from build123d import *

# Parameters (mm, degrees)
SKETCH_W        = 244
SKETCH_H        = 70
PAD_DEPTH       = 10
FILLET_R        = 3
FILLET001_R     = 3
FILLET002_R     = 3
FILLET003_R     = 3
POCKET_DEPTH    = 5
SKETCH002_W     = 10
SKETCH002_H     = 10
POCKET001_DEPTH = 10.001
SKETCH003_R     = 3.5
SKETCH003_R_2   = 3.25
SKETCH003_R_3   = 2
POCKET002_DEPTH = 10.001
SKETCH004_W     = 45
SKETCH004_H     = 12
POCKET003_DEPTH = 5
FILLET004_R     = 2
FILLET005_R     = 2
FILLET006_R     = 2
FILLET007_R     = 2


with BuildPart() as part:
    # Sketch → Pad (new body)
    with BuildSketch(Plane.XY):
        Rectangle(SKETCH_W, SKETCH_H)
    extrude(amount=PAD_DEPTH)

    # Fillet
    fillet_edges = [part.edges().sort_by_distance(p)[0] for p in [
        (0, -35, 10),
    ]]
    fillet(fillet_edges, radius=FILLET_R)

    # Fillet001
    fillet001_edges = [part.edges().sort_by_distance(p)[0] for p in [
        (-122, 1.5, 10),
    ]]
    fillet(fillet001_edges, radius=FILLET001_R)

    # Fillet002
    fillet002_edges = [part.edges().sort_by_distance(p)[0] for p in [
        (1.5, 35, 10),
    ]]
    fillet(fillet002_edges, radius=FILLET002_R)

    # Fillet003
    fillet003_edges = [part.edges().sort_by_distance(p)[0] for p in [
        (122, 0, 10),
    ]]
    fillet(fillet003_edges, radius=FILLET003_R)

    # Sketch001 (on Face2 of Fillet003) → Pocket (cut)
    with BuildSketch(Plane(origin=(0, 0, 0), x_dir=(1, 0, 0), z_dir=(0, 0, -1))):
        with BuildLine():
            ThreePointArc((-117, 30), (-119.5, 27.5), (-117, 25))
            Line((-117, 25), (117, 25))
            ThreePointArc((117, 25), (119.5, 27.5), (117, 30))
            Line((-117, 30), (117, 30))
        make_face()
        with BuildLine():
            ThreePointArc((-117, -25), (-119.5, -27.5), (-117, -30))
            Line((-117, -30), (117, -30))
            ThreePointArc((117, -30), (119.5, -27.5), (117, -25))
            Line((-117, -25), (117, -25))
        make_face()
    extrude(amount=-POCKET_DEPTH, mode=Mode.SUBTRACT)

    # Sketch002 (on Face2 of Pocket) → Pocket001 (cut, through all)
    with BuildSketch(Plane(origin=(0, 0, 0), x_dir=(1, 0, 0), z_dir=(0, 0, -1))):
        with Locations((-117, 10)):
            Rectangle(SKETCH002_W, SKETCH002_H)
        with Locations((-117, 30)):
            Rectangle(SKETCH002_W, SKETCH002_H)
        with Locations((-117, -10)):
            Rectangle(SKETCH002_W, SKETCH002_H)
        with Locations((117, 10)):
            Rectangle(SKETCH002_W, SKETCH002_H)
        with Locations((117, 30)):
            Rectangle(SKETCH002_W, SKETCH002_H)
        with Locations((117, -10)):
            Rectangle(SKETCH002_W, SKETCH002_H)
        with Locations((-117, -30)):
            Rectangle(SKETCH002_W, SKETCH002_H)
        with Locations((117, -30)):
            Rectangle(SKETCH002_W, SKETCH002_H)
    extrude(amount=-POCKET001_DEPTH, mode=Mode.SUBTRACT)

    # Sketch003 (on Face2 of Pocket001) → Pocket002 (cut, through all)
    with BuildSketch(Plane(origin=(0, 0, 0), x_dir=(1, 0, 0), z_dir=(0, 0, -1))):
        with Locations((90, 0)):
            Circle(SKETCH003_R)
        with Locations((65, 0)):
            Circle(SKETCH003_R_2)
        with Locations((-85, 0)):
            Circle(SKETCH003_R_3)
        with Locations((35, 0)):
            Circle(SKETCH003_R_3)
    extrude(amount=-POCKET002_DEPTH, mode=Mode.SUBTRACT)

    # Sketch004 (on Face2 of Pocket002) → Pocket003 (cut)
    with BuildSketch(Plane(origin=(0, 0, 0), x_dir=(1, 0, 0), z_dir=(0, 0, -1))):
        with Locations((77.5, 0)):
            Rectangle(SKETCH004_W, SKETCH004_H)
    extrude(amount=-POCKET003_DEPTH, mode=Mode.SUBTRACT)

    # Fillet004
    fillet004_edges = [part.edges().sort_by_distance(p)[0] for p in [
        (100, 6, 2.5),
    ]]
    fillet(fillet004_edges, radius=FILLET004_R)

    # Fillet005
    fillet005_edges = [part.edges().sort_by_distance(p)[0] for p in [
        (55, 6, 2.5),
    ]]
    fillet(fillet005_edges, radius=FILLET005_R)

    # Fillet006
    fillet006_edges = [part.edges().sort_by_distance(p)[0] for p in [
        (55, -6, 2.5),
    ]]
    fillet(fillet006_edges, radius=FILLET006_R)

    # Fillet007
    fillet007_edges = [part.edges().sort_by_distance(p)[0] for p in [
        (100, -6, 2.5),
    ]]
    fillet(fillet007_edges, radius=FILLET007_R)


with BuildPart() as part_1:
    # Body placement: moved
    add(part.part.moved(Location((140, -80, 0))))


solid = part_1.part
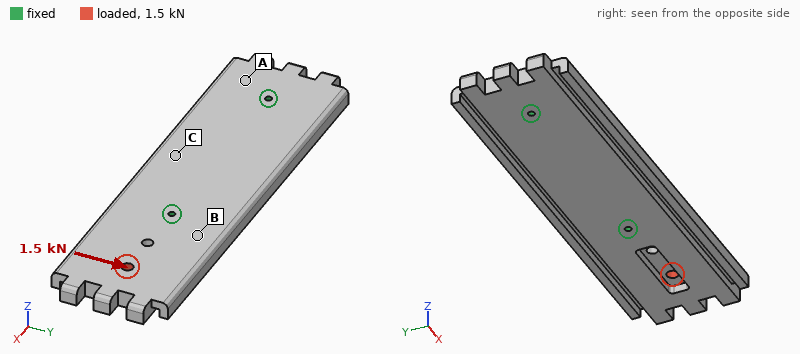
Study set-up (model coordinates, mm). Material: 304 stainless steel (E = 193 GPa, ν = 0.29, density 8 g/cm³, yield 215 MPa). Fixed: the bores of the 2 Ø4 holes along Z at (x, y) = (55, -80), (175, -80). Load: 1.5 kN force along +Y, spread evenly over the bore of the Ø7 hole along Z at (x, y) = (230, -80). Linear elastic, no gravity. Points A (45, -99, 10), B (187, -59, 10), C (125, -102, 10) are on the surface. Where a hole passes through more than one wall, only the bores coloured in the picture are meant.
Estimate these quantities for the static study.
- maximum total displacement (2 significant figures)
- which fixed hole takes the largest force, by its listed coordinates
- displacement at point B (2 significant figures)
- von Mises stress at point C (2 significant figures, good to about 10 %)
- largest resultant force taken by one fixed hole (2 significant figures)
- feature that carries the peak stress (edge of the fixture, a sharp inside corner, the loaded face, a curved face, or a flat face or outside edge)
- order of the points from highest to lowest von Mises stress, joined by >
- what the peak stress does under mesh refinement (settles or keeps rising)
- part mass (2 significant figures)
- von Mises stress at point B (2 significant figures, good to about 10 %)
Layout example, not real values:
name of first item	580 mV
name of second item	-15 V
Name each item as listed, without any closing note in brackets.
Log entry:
maximum total displacement	15 µm
which fixed hole takes the largest force, by its listed coordinates	(175, -80)
displacement at point B	3.6 µm
von Mises stress at point C	4.3 MPa
largest resultant force taken by one fixed hole	2.2 kN
feature that carries the peak stress	edge of the fixture
order of the points from highest to lowest von Mises stress, joined by >	B > C > A
what the peak stress does under mesh refinement	keeps rising
part mass	1.2 kg
von Mises stress at point B	7.7 MPa
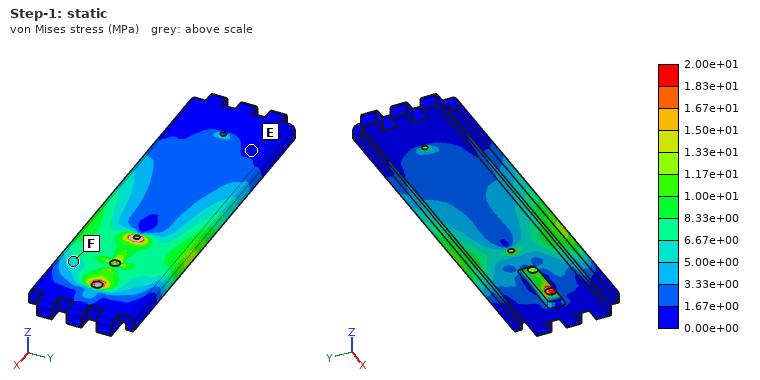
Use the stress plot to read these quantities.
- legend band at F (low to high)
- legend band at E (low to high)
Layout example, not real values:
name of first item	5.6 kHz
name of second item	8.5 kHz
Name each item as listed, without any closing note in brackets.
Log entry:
legend band at F	5.00e+00 to 6.67e+00 MPa
legend band at E	0.00e+00 to 1.67e+00 MPa
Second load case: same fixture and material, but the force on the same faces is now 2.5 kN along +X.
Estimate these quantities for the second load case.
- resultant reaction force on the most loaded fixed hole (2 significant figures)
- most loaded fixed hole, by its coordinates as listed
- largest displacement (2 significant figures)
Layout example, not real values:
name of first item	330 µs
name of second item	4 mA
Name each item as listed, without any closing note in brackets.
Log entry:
resultant reaction force on the most loaded fixed hole	2.0 kN
most loaded fixed hole, by its coordinates as listed	(175, -80)
largest displacement	24 µm
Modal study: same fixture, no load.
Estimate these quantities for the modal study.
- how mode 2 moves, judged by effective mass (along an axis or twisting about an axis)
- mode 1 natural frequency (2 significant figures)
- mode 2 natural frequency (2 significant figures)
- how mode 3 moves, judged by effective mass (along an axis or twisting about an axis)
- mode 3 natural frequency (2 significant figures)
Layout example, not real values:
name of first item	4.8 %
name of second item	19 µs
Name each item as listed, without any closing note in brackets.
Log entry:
how mode 2 moves, judged by effective mass	twisting about X
mode 1 natural frequency	970 Hz
mode 2 natural frequency	2000 Hz
how mode 3 moves, judged by effective mass	along Z
mode 3 natural frequency	2500 Hz
